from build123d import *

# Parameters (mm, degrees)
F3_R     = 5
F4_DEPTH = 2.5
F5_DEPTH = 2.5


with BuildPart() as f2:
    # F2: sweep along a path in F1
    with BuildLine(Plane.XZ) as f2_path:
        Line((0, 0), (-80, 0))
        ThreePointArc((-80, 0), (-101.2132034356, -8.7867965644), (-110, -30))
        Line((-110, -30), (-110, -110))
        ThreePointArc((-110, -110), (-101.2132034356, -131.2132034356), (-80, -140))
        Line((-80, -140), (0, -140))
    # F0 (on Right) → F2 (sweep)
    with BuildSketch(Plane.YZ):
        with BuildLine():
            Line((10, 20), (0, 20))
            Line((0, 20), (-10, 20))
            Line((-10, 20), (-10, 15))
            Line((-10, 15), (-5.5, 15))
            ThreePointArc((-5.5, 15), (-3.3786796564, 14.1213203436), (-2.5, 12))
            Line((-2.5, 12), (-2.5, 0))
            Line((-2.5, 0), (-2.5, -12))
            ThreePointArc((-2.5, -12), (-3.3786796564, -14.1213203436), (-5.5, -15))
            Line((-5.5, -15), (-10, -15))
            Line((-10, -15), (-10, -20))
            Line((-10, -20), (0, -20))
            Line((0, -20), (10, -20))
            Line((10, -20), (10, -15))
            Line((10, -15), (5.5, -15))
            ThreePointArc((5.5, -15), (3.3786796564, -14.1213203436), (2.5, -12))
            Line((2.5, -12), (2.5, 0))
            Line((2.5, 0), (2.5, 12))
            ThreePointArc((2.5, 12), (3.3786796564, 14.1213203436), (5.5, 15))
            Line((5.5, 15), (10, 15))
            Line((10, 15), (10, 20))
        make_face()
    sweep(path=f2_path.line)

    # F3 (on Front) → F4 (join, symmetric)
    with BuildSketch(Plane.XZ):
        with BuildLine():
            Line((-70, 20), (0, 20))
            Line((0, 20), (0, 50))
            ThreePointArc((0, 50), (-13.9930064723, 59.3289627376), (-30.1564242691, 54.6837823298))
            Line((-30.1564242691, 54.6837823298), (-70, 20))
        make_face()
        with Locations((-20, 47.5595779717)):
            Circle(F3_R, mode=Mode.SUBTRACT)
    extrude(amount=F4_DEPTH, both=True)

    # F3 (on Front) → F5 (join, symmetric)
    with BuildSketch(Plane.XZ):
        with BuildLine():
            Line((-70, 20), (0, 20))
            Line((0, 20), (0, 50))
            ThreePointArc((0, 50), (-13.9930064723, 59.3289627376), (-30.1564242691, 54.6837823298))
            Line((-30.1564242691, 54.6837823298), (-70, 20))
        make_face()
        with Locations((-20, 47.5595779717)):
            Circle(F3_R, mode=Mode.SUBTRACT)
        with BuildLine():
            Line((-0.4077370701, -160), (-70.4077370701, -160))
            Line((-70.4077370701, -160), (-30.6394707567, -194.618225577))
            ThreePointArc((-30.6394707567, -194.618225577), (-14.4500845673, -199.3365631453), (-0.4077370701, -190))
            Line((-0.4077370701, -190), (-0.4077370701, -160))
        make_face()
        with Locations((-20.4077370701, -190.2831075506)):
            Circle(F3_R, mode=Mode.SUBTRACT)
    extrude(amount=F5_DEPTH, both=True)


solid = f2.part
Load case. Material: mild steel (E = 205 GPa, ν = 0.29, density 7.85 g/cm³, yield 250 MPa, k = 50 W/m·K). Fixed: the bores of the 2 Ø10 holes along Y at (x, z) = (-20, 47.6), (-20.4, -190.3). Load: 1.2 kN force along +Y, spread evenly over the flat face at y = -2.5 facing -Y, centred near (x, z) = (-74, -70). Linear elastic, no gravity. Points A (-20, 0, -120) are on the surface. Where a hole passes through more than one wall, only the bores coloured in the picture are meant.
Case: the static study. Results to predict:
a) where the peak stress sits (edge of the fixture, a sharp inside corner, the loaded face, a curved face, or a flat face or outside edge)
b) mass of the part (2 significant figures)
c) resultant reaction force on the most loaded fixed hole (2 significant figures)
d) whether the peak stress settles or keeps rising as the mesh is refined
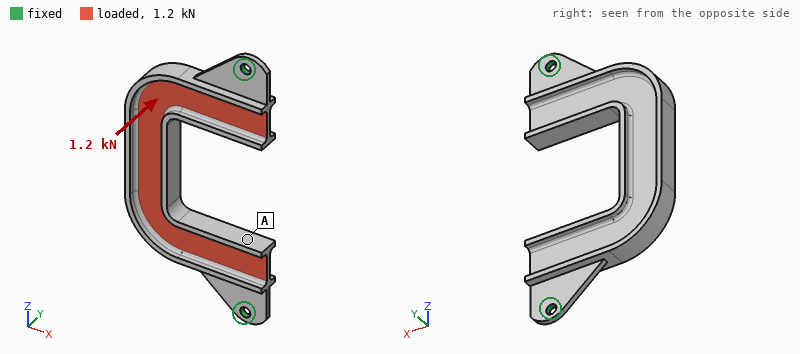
edge of the fixture
1.1 kg
610 N
keeps rising
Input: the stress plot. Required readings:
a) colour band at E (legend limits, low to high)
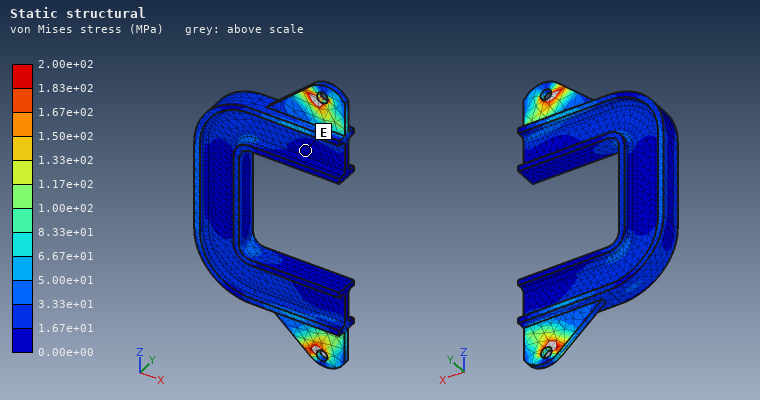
0.00e+00 to 1.67e+01 MPa
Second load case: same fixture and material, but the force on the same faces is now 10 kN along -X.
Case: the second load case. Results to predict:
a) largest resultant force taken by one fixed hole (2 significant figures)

5.8 kN
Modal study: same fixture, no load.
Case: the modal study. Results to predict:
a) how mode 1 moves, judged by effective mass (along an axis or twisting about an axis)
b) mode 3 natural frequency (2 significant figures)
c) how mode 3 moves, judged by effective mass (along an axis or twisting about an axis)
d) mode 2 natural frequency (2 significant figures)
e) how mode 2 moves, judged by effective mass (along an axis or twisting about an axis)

along Y
900 Hz
along Y
730 Hz
twisting about X
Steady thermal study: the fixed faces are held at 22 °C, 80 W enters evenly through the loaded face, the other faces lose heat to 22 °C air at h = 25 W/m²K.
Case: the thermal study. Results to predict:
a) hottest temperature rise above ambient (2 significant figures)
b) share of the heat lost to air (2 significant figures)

68 K
71 %
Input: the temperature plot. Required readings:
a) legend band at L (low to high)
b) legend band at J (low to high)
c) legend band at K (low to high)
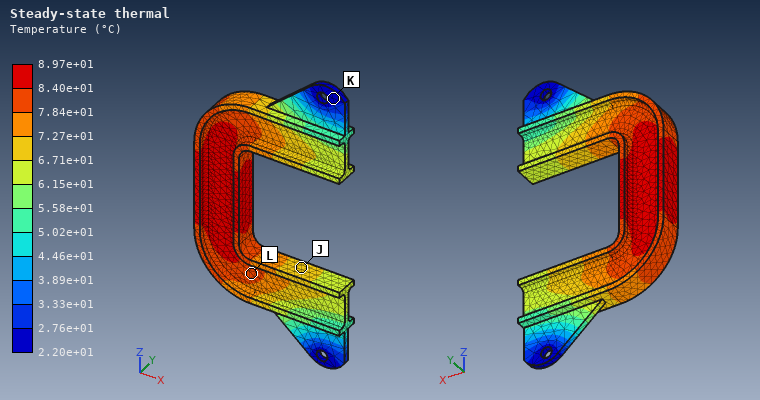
7.84e+01 to 8.40e+01 °C
6.71e+01 to 7.27e+01 °C
2.20e+01 to 2.76e+01 °C
